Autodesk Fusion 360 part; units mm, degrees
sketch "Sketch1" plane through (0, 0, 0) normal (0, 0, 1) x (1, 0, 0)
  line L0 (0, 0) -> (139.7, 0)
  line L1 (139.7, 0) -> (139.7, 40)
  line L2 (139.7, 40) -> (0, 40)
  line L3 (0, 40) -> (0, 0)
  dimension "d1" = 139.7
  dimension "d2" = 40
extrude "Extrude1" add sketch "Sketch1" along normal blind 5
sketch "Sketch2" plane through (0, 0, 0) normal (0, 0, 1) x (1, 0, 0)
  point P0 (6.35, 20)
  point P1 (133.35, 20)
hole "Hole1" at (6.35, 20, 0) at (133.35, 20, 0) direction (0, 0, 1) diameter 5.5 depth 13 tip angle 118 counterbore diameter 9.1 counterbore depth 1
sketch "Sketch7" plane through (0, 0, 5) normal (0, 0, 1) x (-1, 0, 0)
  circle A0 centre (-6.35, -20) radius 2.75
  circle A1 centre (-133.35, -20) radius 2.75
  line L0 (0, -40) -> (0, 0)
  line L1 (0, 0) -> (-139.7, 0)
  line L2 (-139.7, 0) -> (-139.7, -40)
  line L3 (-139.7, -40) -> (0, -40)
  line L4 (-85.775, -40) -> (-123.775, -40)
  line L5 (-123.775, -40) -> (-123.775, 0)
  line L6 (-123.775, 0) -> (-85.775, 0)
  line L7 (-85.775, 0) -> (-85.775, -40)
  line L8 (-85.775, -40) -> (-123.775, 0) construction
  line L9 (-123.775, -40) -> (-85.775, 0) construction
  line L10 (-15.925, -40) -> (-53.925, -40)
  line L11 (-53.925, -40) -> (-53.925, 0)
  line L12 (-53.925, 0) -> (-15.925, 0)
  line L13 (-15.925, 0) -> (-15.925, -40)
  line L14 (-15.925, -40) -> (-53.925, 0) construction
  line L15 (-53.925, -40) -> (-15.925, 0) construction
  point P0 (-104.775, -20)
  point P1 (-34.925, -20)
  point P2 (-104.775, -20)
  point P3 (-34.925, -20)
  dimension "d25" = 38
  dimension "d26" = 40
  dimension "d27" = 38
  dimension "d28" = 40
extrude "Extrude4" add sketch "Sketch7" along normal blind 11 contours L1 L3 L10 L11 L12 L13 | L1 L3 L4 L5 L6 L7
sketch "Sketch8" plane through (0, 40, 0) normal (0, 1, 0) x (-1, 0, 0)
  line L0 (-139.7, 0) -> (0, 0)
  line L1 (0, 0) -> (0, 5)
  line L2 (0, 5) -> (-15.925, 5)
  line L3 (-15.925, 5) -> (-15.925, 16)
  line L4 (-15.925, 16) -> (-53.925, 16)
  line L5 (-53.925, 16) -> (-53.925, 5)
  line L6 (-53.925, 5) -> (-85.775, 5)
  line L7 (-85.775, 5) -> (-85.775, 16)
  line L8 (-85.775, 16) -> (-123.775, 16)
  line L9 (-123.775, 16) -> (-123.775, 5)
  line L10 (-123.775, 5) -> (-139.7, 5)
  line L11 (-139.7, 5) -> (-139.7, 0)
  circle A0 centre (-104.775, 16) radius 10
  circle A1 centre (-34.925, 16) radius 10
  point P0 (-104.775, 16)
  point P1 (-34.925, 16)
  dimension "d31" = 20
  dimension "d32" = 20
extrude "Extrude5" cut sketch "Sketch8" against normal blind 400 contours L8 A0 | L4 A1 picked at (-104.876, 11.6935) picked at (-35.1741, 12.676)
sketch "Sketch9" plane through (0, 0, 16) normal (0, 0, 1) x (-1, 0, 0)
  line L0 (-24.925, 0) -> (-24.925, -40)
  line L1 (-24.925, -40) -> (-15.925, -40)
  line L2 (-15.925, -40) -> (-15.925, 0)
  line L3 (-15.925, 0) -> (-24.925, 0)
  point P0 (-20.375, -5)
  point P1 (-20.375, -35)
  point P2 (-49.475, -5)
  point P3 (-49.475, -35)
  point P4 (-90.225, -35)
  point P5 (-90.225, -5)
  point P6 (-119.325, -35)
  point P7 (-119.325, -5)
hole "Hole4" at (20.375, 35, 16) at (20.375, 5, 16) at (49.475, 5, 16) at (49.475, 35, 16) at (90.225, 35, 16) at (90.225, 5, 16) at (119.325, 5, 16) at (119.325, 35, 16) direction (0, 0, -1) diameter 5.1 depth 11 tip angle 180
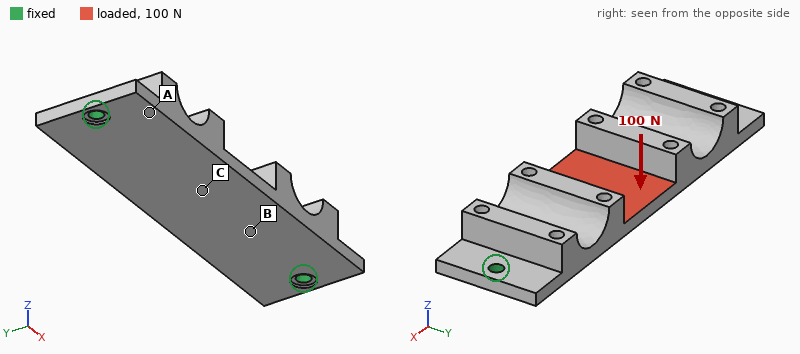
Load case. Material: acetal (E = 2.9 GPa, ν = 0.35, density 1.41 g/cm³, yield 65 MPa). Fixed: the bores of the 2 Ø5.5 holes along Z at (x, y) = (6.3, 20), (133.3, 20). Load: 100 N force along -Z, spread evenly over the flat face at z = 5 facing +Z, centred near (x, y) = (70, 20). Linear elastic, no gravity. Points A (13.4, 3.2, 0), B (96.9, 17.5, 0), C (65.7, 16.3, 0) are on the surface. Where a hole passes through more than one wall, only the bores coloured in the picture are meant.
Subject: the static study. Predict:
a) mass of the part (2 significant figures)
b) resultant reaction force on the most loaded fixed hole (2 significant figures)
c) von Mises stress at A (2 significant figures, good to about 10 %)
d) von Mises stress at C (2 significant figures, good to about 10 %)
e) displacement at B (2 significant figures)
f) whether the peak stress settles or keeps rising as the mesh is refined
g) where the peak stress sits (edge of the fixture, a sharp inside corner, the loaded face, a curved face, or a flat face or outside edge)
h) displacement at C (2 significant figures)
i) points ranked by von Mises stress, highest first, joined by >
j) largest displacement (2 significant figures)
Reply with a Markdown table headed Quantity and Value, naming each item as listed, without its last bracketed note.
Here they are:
| Quantity | Value |
|---|---|
| mass of the part | 66 g |
| resultant reaction force on the most loaded fixed hole | 58 N |
| von Mises stress at A | 4.5 MPa |
| von Mises stress at C | 7.2 MPa |
| displacement at B | 0.56 mm |
| whether the peak stress settles or keeps rising as the mesh is refined | keeps rising |
| where the peak stress sits | edge of the fixture |
| displacement at C | 0.86 mm |
| points ranked by von Mises stress, highest first, joined by > | C > A > B |
| largest displacement | 0.90 mm |
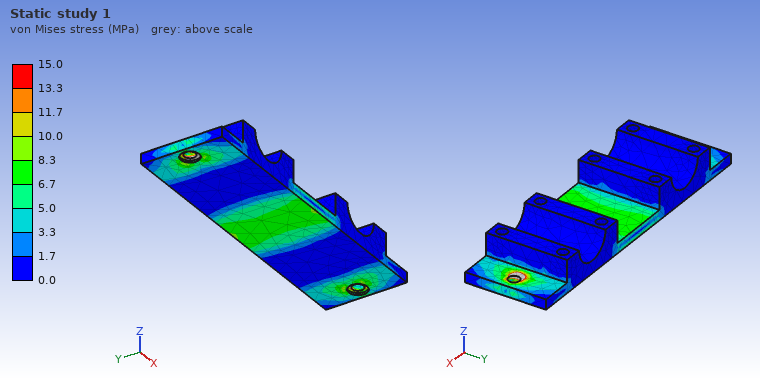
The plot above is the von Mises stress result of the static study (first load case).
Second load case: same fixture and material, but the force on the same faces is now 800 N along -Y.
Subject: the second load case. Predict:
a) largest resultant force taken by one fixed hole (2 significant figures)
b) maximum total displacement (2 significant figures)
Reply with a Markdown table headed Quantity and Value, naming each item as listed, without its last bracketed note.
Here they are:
| Quantity | Value |
|---|---|
| largest resultant force taken by one fixed hole | 400 N |
| maximum total displacement | 0.50 mm |
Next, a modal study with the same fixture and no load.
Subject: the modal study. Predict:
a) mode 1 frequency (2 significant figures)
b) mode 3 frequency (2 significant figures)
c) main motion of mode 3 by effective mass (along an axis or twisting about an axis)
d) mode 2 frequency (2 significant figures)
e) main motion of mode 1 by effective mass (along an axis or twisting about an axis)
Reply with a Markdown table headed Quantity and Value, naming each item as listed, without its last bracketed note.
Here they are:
| Quantity | Value |
|---|---|
| mode 1 frequency | 340 Hz |
| mode 3 frequency | 1100 Hz |
| main motion of mode 3 by effective mass | twisting about Y |
| mode 2 frequency | 730 Hz |
| main motion of mode 1 by effective mass | along Z |
